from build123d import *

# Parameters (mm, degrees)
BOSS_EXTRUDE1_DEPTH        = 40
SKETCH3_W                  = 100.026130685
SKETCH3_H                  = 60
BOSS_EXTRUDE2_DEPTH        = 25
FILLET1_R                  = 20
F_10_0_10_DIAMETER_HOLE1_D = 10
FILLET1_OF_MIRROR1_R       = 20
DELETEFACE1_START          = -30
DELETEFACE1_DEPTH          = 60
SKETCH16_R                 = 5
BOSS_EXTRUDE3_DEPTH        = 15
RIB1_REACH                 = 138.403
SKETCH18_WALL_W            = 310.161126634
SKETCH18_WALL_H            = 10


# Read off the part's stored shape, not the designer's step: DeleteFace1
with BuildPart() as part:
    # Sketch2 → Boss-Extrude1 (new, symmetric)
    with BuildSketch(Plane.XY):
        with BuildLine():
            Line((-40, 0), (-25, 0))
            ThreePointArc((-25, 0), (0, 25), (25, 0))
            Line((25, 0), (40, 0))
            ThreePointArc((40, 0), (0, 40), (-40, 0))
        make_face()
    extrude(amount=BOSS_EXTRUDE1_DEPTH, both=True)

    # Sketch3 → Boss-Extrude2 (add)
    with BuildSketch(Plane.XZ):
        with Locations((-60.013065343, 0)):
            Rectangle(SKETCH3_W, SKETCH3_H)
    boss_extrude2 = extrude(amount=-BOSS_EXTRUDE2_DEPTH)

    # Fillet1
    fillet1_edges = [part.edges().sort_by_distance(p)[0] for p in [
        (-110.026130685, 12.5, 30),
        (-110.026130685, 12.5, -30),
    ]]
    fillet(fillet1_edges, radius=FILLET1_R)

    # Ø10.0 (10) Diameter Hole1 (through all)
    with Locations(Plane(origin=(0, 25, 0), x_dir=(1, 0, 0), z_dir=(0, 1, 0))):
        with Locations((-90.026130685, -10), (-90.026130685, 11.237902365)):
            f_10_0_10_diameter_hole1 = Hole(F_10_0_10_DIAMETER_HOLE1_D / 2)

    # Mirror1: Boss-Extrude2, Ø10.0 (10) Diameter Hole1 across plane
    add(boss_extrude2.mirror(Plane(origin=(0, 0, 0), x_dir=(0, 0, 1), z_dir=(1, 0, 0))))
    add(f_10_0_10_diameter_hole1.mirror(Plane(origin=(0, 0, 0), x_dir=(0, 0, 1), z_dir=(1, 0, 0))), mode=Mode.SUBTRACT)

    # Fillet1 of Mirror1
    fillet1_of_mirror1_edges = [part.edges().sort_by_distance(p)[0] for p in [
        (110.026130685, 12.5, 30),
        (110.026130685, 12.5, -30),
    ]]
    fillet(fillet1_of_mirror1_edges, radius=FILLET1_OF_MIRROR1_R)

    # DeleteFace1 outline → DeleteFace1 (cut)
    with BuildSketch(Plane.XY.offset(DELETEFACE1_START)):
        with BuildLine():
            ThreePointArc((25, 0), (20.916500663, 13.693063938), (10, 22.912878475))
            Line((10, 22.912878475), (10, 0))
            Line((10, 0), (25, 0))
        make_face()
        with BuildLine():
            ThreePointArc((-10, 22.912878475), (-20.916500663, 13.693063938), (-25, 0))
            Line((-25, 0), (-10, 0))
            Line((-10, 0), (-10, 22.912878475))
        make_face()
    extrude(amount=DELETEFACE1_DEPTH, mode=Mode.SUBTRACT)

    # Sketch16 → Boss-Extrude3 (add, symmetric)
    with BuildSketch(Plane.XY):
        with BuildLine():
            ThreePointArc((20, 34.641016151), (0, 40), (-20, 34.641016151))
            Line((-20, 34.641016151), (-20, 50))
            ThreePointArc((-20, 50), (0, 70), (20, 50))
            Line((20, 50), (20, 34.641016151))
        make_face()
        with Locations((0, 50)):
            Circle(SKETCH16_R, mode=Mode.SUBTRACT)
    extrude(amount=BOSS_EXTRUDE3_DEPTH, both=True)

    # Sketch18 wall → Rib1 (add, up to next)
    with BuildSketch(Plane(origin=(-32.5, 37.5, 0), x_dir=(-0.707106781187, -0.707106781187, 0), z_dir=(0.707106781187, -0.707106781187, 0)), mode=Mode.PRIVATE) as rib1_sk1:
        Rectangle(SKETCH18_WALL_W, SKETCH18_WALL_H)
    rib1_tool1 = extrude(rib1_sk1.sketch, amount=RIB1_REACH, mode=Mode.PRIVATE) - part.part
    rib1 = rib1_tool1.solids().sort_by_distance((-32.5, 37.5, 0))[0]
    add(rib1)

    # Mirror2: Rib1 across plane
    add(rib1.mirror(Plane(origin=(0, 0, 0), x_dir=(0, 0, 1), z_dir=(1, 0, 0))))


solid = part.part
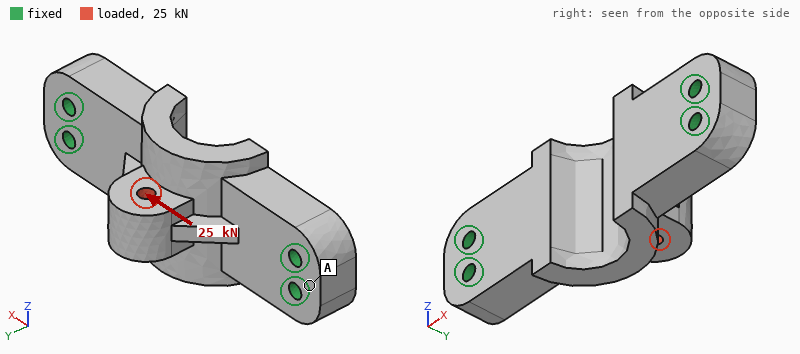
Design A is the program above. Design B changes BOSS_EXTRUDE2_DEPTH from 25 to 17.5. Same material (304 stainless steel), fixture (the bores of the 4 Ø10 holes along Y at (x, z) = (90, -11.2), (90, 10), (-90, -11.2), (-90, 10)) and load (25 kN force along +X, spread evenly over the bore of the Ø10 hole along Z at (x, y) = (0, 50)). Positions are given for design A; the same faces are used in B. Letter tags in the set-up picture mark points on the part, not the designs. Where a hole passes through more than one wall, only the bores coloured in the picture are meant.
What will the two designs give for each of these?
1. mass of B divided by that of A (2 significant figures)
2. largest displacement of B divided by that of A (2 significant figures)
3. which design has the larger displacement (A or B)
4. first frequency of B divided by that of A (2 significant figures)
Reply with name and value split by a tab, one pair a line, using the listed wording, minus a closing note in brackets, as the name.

mass of B divided by that of A	0.83
largest displacement of B divided by that of A	1.5
which design has the larger displacement	B
first frequency of B divided by that of A	0.69
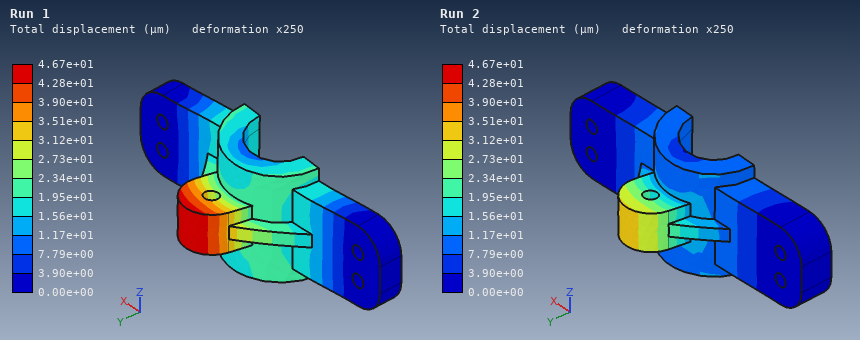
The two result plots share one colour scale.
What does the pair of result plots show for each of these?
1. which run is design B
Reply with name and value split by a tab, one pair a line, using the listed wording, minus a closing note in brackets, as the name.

which run is design B	Run 1
